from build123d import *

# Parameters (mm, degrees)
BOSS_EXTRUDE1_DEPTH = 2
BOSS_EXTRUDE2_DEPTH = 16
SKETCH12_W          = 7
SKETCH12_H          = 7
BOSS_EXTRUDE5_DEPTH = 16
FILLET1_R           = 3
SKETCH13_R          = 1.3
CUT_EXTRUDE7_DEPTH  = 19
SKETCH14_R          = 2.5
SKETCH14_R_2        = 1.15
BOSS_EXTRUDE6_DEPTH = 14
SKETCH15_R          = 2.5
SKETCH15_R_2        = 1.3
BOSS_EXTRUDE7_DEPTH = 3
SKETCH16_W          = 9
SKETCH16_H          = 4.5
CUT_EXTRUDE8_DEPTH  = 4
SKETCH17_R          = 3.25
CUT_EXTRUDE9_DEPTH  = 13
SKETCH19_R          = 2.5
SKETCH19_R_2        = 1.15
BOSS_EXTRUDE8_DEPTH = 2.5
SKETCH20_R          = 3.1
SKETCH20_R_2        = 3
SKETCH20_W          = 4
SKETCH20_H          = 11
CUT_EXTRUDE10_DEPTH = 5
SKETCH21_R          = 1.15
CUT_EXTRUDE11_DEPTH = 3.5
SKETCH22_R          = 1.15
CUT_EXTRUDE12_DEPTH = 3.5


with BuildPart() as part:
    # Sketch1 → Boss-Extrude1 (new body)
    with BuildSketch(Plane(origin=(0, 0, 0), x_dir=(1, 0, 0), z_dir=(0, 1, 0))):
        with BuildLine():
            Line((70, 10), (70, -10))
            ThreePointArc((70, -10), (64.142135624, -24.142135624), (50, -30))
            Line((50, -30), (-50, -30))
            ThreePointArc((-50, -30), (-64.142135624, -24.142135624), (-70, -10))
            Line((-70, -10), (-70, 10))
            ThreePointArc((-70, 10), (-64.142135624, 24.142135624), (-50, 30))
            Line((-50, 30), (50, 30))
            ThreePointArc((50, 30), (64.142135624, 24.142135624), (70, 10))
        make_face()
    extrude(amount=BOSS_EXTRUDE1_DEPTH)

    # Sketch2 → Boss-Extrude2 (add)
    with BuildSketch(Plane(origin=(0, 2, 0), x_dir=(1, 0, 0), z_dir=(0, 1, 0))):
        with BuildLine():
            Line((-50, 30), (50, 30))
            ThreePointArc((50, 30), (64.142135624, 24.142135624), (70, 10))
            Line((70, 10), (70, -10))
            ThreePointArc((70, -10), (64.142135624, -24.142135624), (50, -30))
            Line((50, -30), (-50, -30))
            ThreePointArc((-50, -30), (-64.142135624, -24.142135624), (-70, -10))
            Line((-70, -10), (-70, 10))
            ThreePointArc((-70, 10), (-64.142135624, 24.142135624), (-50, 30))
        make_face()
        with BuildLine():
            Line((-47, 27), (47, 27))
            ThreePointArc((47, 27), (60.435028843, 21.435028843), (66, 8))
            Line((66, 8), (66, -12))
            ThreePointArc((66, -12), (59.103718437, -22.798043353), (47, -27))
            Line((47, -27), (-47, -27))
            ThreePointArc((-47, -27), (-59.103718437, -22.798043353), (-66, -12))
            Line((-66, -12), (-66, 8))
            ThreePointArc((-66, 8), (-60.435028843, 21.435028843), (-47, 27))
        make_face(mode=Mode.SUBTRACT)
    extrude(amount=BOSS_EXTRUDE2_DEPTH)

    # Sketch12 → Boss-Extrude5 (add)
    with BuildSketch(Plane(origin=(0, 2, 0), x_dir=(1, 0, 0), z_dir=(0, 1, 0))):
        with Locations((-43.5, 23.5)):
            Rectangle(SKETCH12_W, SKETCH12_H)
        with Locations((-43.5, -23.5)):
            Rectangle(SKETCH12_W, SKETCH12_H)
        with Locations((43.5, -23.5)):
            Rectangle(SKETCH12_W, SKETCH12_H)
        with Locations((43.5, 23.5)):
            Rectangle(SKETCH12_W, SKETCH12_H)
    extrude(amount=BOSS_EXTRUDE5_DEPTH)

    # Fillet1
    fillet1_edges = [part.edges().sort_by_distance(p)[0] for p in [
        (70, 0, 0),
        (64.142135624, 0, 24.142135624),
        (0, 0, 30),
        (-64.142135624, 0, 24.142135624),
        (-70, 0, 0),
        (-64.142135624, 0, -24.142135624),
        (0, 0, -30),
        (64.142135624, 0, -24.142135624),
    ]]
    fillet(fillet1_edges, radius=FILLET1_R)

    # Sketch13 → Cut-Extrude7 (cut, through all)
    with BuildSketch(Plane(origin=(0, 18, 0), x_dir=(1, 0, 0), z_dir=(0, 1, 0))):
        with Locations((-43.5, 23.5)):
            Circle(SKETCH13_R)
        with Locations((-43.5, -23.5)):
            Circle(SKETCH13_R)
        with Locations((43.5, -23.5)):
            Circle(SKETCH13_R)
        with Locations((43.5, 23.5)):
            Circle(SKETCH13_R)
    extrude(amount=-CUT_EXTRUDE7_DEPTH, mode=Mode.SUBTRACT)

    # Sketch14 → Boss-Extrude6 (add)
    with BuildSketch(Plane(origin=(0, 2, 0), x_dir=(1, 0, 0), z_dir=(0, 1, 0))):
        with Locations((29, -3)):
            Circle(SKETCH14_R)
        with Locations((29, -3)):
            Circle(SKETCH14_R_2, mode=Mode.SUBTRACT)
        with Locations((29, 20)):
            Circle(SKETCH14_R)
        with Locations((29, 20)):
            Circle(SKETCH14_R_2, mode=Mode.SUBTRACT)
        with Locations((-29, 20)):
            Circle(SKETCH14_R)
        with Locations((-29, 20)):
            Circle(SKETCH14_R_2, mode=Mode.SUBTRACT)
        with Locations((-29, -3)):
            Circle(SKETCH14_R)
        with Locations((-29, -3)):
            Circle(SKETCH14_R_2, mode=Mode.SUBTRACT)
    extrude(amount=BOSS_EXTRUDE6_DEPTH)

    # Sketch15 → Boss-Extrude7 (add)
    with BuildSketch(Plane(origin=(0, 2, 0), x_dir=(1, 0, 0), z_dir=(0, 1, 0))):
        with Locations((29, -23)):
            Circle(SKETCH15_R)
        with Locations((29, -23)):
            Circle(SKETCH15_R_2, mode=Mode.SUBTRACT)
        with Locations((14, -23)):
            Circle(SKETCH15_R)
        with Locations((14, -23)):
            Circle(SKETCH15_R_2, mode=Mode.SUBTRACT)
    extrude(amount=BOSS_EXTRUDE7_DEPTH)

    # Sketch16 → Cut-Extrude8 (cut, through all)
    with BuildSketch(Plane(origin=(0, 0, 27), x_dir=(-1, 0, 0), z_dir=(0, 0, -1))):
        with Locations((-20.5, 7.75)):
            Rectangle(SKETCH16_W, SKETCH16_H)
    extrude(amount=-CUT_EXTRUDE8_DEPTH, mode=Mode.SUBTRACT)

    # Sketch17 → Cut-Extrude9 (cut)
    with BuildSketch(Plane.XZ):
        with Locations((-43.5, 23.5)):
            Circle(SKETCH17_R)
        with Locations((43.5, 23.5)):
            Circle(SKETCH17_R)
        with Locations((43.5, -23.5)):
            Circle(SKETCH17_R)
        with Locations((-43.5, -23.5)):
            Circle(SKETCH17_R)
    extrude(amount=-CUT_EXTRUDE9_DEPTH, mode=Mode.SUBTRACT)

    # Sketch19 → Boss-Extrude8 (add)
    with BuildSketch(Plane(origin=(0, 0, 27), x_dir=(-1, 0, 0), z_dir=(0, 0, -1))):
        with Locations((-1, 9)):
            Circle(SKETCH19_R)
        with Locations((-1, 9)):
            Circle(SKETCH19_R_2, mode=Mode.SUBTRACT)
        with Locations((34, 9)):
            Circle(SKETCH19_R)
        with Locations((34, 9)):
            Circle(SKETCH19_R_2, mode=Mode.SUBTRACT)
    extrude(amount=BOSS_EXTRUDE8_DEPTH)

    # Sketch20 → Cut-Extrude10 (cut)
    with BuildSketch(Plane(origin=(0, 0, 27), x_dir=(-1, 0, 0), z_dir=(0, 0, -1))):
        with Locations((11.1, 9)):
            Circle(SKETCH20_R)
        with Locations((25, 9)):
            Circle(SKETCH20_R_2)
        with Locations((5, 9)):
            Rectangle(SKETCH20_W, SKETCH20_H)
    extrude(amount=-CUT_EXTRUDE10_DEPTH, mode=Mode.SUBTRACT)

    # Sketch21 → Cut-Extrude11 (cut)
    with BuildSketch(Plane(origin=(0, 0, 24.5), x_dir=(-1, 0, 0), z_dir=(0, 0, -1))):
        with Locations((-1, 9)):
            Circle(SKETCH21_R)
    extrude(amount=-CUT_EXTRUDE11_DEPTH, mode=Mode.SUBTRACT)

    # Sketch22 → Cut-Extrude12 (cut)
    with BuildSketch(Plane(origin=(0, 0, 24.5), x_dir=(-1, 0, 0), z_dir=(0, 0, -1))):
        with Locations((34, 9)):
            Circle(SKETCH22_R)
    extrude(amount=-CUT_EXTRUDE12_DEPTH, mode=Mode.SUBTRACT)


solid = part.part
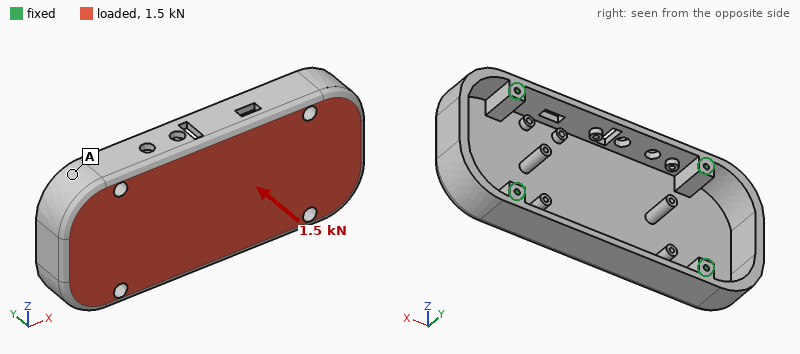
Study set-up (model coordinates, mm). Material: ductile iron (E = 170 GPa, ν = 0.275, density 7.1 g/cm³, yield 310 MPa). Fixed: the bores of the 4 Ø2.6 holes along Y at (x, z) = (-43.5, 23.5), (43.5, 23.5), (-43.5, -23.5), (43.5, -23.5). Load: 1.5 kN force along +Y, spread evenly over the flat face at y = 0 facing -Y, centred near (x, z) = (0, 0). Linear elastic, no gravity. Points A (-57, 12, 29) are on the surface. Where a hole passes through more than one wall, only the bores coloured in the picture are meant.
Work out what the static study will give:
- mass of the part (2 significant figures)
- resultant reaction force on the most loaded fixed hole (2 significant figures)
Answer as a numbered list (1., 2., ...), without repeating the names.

1. 260 g
2. 410 N
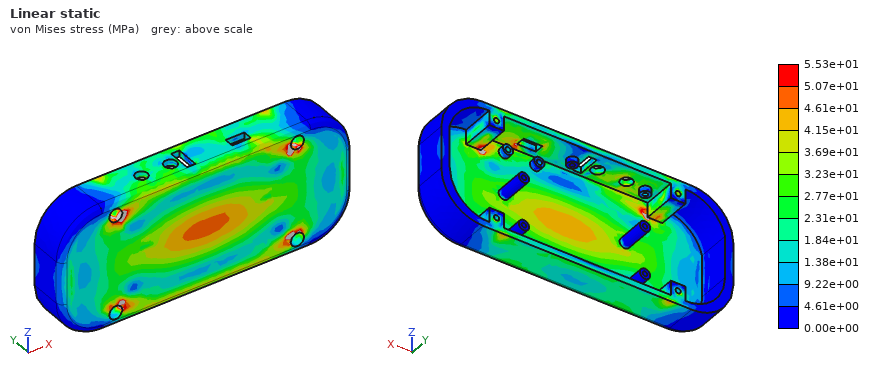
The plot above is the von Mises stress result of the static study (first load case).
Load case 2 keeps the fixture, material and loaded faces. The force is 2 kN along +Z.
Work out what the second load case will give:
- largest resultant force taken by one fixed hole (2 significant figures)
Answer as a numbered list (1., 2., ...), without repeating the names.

1. 530 N
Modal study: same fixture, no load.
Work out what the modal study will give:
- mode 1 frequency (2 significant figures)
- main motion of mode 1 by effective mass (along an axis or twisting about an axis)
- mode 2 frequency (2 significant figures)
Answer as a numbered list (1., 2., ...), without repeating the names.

1. 2500 Hz
2. along Y
3. 4000 Hz
